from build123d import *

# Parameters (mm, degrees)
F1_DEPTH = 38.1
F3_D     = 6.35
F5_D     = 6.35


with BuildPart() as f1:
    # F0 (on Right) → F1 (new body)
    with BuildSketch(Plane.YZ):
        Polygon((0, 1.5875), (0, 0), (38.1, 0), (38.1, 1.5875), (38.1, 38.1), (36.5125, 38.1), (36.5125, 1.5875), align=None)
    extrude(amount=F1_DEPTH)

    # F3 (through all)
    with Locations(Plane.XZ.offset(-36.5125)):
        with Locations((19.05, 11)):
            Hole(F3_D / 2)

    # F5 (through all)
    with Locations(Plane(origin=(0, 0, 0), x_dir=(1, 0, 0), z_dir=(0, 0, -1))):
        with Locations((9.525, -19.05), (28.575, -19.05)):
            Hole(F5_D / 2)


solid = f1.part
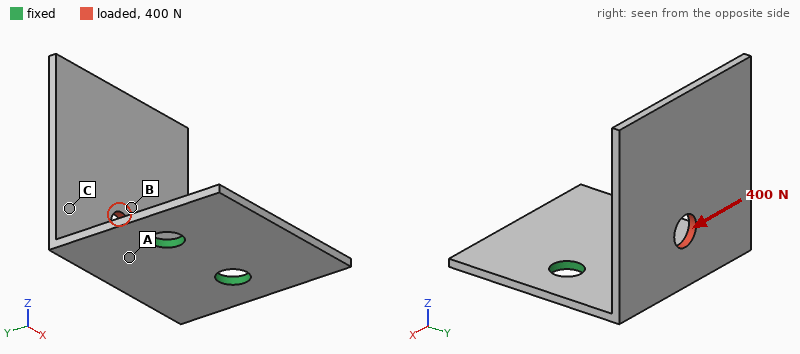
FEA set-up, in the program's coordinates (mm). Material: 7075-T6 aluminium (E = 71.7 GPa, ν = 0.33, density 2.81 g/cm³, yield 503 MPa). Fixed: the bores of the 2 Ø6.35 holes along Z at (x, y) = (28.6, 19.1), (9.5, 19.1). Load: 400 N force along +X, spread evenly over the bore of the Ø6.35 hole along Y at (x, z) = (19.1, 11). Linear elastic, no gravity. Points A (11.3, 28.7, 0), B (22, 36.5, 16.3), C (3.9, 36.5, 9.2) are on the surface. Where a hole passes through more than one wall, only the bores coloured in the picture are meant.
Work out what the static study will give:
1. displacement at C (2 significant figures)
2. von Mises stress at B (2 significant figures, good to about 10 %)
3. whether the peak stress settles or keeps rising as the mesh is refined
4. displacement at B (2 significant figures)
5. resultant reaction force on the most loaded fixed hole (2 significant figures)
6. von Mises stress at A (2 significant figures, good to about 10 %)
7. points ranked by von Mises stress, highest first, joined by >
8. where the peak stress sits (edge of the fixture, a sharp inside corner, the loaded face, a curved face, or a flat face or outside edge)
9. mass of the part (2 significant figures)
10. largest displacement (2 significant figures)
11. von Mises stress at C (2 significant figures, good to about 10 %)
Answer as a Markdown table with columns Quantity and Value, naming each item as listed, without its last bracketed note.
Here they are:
| Quantity | Value |
|---|---|
| displacement at C | 0.32 mm |
| von Mises stress at B | 17 MPa |
| whether the peak stress settles or keeps rising as the mesh is refined | keeps rising |
| displacement at B | 0.30 mm |
| resultant reaction force on the most loaded fixed hole | 390 N |
| von Mises stress at A | 96 MPa |
| points ranked by von Mises stress, highest first, joined by > | A > C > B |
| where the peak stress sits | edge of the fixture |
| mass of the part | 12 g |
| largest displacement | 0.79 mm |
| von Mises stress at C | 57 MPa |
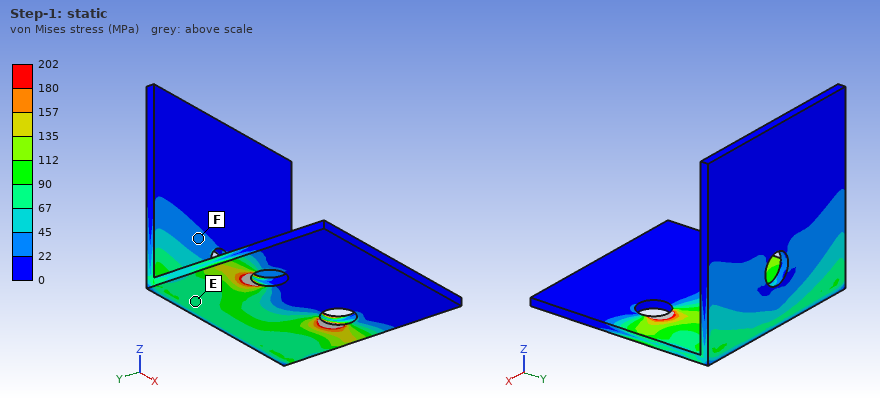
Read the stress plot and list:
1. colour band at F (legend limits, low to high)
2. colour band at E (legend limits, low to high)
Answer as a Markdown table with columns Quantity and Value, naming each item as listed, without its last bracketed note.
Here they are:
| Quantity | Value |
|---|---|
| colour band at F | 22 to 45 MPa |
| colour band at E | 67 to 90 MPa |
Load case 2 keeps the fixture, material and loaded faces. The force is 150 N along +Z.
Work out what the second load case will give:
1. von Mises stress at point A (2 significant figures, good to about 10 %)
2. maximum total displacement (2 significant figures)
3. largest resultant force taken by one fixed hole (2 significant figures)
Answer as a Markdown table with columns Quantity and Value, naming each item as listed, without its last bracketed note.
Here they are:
| Quantity | Value |
|---|---|
| von Mises stress at point A | 72 MPa |
| maximum total displacement | 0.79 mm |
| largest resultant force taken by one fixed hole | 75 N |
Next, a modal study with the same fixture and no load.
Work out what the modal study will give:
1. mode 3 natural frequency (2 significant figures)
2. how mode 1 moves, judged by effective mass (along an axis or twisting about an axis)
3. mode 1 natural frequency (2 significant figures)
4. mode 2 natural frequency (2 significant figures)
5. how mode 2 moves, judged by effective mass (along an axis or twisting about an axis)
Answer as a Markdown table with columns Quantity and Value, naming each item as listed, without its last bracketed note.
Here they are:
| Quantity | Value |
|---|---|
| mode 3 natural frequency | 2100 Hz |
| how mode 1 moves, judged by effective mass | along Y |
| mode 1 natural frequency | 560 Hz |
| mode 2 natural frequency | 1200 Hz |
| how mode 2 moves, judged by effective mass | along X |
